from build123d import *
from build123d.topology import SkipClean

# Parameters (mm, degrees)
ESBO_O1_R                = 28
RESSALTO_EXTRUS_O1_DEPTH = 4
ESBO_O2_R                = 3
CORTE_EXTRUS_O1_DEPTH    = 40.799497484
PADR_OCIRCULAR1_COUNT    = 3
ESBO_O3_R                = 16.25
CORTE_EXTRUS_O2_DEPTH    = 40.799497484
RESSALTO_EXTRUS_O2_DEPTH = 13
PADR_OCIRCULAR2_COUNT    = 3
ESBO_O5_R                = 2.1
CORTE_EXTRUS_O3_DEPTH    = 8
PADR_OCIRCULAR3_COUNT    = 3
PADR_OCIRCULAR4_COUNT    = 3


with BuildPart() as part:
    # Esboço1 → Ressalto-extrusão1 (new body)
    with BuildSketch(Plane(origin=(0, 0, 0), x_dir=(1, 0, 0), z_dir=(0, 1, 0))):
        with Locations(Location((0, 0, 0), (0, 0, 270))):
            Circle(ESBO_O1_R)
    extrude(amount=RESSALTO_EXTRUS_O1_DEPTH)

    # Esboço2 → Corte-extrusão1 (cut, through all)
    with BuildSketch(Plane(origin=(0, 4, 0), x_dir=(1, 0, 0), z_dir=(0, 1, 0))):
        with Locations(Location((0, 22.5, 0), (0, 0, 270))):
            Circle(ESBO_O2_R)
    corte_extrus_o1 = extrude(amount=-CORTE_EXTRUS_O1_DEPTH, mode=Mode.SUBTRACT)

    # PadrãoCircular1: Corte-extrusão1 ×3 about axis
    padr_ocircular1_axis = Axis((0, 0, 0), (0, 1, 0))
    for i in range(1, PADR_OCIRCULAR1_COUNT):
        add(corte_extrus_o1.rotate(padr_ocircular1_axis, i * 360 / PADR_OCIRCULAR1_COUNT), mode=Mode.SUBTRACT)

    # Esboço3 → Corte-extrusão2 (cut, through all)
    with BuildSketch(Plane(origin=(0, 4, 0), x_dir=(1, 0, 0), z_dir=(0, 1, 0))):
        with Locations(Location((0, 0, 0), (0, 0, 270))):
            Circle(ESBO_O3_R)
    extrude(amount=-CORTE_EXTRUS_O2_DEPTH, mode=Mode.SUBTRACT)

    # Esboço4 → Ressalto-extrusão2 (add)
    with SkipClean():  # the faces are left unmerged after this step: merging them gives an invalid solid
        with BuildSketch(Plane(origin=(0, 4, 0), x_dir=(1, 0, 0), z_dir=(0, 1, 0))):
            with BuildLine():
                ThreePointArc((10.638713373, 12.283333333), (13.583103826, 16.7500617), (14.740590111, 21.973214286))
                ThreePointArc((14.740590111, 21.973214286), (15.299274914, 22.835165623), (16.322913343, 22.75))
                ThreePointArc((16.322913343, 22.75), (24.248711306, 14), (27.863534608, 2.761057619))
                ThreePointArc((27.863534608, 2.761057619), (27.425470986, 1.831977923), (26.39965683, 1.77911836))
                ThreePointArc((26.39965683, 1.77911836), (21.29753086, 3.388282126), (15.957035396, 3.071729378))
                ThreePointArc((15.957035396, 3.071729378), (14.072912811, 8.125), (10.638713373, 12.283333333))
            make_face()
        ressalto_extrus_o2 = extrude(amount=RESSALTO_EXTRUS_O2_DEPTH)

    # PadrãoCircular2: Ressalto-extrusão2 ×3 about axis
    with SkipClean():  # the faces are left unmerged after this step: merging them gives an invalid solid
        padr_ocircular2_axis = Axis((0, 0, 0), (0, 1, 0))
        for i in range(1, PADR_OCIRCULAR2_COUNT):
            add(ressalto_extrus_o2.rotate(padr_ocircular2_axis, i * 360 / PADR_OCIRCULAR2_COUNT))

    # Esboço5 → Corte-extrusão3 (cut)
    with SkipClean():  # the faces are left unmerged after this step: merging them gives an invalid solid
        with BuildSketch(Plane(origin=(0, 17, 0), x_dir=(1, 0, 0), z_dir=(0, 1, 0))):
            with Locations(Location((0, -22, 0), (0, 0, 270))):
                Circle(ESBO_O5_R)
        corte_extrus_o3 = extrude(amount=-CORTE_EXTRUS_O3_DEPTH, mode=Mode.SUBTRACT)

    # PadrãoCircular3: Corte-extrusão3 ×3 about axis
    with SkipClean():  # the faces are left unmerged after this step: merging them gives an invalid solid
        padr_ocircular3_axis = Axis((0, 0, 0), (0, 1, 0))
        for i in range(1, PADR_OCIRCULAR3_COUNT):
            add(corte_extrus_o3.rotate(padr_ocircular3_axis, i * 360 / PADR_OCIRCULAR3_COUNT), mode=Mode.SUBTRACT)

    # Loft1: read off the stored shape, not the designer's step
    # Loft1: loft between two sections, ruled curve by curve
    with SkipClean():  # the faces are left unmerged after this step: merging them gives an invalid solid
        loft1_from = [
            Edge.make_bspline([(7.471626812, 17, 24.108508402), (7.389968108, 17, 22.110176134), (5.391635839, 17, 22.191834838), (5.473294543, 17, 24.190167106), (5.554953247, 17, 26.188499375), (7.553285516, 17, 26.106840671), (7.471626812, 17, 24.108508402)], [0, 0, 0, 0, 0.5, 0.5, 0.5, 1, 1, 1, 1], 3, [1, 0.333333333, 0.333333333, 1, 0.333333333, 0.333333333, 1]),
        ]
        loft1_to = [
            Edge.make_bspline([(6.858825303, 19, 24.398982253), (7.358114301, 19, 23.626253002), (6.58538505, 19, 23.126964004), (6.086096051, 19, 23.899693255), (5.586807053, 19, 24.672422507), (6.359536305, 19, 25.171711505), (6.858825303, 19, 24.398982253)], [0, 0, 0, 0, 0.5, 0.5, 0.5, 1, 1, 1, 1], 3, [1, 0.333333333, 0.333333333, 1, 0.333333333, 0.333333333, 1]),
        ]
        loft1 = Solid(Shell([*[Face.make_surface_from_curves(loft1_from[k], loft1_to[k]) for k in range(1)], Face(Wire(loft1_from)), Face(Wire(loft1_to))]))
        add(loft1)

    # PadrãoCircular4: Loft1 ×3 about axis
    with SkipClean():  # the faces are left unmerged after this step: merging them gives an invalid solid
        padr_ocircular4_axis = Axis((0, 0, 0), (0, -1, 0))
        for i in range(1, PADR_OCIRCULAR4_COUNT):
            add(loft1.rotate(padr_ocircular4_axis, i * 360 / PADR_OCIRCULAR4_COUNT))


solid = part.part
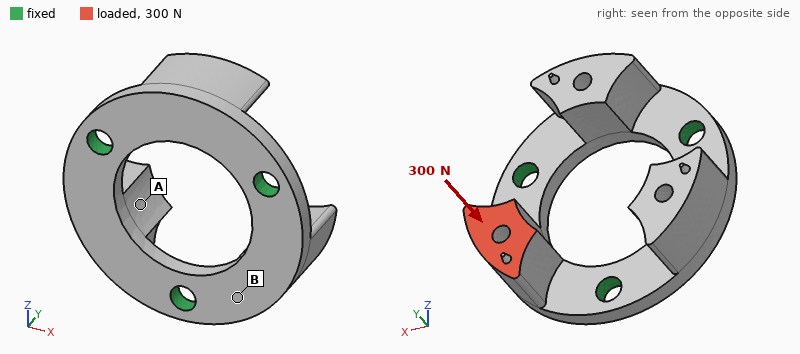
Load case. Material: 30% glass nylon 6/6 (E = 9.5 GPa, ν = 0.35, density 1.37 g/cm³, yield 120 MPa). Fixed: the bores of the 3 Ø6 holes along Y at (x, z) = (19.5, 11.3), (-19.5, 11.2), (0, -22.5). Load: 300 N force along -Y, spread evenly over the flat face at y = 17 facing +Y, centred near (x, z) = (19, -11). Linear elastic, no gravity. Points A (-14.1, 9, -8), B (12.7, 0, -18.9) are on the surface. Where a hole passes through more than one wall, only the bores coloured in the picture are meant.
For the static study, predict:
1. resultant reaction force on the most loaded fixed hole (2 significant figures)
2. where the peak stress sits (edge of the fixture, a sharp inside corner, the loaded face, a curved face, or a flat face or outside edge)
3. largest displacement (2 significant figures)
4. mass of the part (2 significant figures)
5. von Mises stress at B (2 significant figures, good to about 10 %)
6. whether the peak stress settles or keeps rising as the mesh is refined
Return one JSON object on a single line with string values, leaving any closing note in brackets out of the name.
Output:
{"resultant reaction force on the most loaded fixed hole": "150 N", "where the peak stress sits": "edge of the fixture", "largest displacement": "0.31 mm", "mass of the part": "19 g", "von Mises stress at B": "15 MPa", "whether the peak stress settles or keeps rising as the mesh is refined": "keeps rising"}
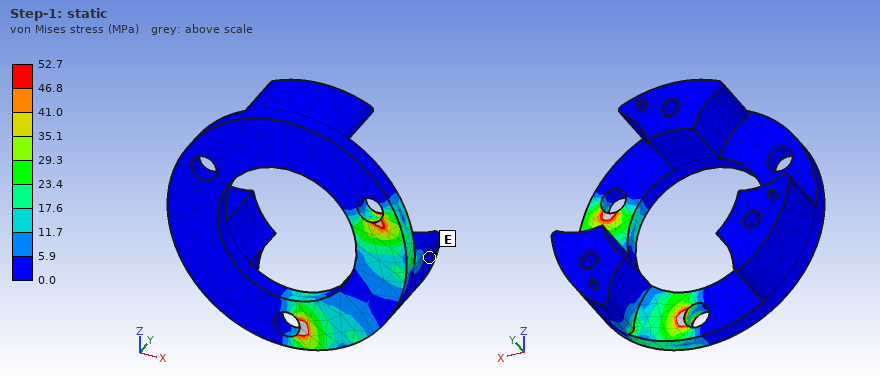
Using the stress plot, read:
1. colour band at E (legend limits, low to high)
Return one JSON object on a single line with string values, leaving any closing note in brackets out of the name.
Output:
{"colour band at E": "0.0 to 5.9 MPa"}
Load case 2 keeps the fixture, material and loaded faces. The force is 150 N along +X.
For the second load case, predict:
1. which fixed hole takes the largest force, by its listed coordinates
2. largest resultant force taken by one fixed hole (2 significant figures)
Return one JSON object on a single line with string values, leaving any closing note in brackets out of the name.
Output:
{"which fixed hole takes the largest force, by its listed coordinates": "(0, -22.5)", "largest resultant force taken by one fixed hole": "140 N"}
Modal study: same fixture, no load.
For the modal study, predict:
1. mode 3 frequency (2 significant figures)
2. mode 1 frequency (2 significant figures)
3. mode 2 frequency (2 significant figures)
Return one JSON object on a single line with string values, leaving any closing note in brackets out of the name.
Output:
{"mode 3 frequency": "2300 Hz", "mode 1 frequency": "2300 Hz", "mode 2 frequency": "2300 Hz"}
